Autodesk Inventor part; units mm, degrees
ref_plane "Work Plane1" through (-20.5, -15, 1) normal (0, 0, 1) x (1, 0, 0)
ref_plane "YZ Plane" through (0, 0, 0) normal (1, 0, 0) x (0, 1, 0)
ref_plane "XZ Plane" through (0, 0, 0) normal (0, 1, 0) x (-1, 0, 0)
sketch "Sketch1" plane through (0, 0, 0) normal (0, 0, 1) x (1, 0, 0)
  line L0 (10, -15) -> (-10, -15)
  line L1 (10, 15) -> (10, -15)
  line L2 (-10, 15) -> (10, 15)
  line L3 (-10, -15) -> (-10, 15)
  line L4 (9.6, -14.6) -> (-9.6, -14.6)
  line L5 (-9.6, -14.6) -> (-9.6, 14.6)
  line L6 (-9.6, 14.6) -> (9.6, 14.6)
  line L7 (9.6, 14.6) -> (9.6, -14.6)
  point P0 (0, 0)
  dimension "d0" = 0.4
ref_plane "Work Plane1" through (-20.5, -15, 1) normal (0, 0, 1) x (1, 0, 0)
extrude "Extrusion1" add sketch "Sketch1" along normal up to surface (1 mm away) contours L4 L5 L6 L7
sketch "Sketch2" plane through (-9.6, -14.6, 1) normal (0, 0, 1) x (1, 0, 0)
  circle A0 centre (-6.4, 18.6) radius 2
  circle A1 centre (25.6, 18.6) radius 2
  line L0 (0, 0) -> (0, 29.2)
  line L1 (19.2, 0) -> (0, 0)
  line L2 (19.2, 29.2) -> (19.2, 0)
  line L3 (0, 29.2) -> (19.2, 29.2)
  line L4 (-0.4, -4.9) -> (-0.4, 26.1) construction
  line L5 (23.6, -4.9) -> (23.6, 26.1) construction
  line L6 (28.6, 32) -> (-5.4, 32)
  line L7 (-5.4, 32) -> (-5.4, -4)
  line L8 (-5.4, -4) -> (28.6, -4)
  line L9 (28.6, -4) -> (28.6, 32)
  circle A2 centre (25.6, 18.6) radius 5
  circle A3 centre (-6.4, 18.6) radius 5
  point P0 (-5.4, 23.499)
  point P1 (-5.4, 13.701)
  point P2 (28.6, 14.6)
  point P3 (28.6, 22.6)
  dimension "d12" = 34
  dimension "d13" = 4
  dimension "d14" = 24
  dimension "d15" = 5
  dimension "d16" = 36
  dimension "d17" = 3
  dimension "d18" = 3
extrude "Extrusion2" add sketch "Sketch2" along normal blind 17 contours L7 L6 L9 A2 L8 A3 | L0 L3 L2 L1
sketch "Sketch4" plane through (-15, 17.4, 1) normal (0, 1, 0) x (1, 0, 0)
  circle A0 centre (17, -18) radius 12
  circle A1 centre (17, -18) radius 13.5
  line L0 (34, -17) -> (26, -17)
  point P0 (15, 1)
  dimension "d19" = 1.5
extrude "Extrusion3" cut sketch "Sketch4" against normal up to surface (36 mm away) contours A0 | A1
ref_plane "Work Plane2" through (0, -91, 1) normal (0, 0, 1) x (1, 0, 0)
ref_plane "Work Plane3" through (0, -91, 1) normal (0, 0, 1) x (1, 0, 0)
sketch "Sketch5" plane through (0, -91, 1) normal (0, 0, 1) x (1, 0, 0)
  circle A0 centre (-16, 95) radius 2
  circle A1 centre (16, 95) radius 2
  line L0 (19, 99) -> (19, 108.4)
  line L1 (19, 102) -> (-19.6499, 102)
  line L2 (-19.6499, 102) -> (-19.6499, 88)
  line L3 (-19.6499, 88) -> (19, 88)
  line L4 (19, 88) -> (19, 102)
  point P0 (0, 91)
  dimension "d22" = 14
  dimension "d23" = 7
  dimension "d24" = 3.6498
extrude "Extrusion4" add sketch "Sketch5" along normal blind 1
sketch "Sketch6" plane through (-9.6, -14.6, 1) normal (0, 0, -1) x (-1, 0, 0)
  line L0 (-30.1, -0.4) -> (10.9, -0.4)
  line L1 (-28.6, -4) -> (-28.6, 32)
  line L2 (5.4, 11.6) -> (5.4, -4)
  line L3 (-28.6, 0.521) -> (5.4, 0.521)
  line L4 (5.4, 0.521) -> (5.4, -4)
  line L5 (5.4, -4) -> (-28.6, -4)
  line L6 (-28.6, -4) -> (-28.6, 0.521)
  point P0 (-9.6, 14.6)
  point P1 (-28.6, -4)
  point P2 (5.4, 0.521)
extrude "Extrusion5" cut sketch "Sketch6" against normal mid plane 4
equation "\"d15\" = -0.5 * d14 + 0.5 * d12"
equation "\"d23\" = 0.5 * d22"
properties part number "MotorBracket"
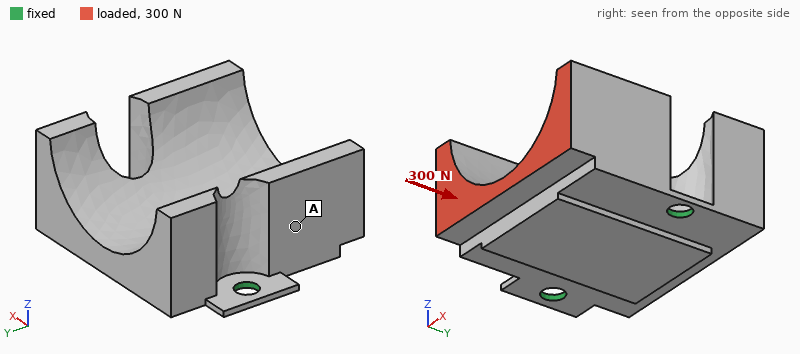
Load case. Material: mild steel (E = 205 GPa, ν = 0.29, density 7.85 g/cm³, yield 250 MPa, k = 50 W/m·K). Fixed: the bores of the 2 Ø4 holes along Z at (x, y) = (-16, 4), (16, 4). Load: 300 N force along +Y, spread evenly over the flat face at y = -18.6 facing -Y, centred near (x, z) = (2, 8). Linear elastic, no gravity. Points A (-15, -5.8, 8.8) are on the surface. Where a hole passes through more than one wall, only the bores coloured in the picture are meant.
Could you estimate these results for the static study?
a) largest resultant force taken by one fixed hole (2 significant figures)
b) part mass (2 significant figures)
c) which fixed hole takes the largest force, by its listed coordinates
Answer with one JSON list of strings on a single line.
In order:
["170 N", "82 g", "(16, 4)"]
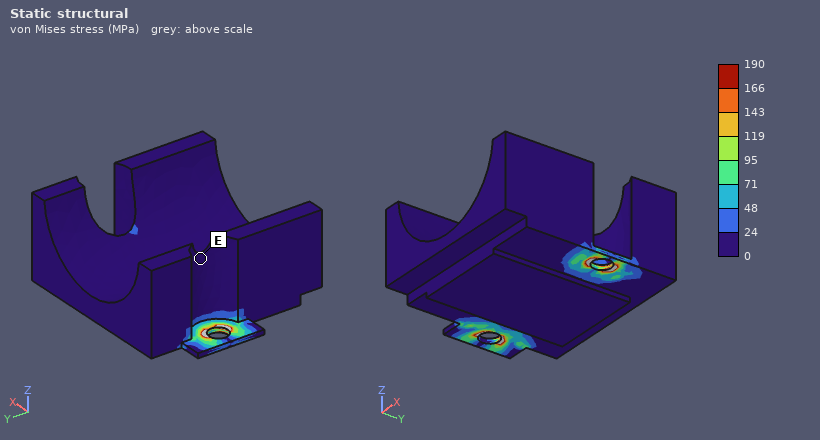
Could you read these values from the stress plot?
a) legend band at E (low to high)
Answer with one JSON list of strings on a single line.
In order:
["0 to 24 MPa"]
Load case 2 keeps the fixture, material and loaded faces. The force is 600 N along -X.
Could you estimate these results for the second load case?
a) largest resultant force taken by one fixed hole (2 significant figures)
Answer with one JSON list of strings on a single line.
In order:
["550 N"]
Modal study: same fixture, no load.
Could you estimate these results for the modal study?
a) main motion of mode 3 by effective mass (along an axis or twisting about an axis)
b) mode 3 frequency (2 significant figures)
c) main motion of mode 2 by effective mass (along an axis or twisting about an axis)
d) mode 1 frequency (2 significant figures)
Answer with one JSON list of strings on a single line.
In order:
["along Z", "6500 Hz", "along Z", "1300 Hz"]
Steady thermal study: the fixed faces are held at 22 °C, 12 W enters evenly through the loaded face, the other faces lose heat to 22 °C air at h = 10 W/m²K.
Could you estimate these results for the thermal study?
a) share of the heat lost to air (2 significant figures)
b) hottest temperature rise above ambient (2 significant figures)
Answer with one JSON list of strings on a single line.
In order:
["13 %", "49 K"]
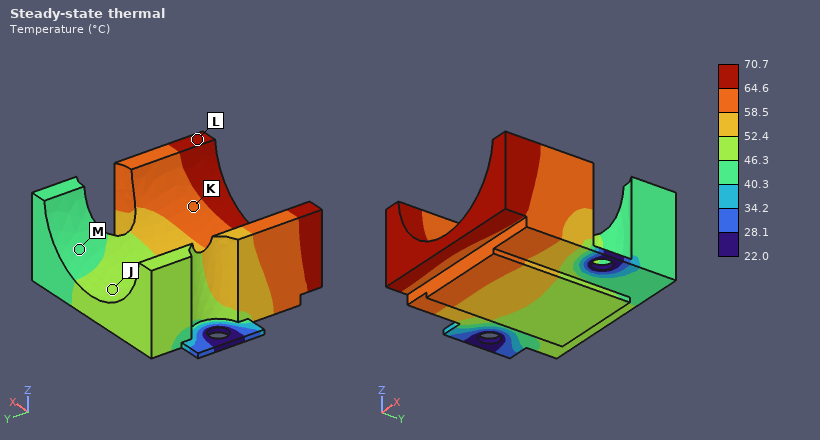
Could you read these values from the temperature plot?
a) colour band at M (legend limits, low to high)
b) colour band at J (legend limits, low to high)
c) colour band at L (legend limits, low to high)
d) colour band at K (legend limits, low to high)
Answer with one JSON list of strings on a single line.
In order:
["40.3 to 46.3 °C", "46.3 to 52.4 °C", "64.6 to 70.7 °C", "58.5 to 64.6 °C"]
